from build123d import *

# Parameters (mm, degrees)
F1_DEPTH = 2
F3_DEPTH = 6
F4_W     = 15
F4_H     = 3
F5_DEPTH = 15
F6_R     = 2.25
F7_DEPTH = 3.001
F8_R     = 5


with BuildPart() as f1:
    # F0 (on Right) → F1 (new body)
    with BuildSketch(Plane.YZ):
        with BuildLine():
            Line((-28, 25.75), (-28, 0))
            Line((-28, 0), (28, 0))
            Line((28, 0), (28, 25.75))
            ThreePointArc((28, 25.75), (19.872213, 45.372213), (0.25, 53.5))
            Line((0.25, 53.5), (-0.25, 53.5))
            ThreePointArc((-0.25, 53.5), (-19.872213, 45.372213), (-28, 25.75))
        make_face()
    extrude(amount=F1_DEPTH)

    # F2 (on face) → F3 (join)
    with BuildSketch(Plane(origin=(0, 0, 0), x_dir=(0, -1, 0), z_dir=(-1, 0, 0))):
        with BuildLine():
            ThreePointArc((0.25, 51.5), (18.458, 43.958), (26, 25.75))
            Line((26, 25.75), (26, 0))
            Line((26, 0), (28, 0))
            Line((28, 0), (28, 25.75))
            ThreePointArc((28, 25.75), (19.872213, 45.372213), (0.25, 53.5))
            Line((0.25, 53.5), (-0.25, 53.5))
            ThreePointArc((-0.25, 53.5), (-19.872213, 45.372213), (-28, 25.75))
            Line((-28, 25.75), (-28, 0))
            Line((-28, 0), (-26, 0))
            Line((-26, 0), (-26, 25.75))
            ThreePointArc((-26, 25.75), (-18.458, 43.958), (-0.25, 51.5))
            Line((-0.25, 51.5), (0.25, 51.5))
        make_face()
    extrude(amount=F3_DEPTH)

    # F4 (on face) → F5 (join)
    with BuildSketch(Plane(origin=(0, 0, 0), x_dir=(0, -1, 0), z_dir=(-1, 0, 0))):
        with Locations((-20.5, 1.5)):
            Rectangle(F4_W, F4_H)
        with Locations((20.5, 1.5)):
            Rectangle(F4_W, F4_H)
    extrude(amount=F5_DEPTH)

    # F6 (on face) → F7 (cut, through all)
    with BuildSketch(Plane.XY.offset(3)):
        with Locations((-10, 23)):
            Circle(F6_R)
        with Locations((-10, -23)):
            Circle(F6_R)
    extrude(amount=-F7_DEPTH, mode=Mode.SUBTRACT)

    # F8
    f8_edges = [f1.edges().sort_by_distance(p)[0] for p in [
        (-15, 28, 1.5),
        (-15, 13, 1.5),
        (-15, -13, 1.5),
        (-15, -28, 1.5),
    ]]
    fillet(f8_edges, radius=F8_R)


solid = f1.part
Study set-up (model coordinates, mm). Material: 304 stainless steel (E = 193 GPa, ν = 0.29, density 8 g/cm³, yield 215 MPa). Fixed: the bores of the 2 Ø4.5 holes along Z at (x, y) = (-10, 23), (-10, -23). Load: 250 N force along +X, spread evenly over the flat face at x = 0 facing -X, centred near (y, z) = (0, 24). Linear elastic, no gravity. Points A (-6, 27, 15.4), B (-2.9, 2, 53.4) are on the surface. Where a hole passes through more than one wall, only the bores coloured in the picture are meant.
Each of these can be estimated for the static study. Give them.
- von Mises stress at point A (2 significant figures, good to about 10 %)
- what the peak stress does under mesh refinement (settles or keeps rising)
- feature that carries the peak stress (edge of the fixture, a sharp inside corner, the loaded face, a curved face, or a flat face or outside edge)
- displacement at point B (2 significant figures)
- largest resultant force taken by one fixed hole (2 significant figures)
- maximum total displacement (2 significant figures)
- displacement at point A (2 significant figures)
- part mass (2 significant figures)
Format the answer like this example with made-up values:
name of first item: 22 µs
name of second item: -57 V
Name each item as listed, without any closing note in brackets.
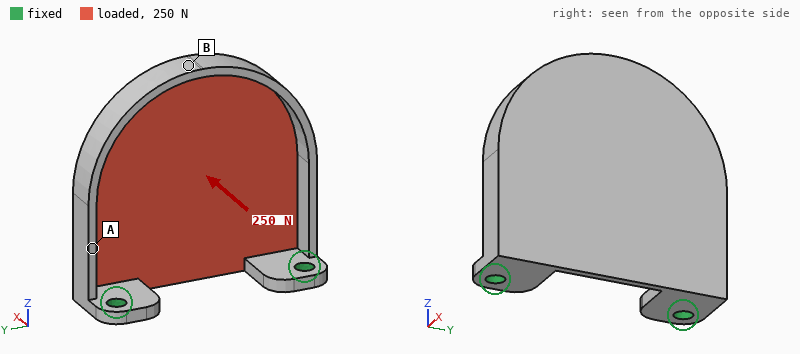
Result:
von Mises stress at point A: 48 MPa
what the peak stress does under mesh refinement: keeps rising
feature that carries the peak stress: edge of the fixture
displacement at point B: 0.22 mm
largest resultant force taken by one fixed hole: 130 N
maximum total displacement: 0.22 mm
displacement at point A: 0.046 mm
part mass: 65 g
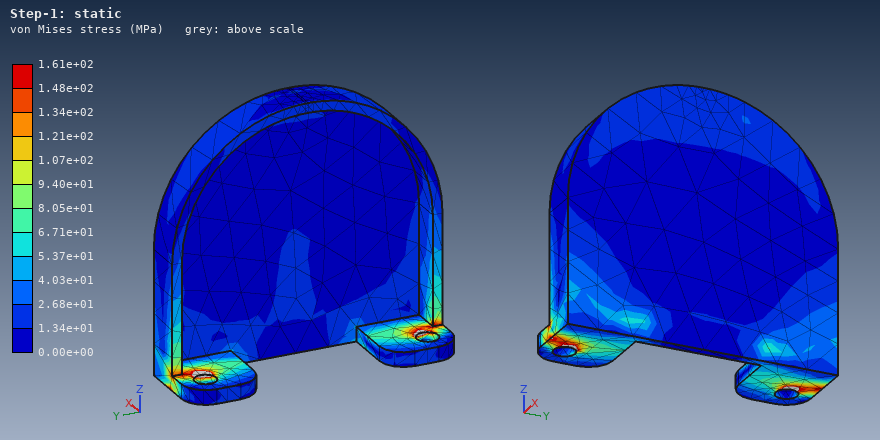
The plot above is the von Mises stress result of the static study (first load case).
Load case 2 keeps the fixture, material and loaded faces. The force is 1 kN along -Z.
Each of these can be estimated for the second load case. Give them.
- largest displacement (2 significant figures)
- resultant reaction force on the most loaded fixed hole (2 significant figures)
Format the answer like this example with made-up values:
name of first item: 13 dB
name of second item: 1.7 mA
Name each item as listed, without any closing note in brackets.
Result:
largest displacement: 0.15 mm
resultant reaction force on the most loaded fixed hole: 500 N
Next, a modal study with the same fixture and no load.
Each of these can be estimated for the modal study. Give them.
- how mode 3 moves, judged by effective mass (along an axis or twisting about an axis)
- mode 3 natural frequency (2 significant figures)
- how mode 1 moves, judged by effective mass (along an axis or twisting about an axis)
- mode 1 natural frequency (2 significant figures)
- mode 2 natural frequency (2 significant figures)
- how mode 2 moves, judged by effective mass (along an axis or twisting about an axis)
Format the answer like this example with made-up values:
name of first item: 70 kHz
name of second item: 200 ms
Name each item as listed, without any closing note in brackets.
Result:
how mode 3 moves, judged by effective mass: along Z
mode 3 natural frequency: 5000 Hz
how mode 1 moves, judged by effective mass: along X
mode 1 natural frequency: 850 Hz
mode 2 natural frequency: 2100 Hz
how mode 2 moves, judged by effective mass: along Y
